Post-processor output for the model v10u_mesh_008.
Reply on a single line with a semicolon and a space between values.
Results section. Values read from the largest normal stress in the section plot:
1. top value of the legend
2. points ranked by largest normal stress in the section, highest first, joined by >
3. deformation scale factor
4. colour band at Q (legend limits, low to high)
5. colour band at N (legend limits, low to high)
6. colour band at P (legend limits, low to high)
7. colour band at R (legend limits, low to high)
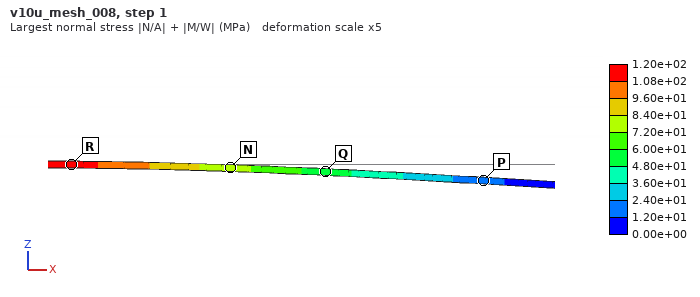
1.20e+02 MPa; R > N > Q > P; 5; 4.80e+01 to 6.00e+01 MPa; 7.20e+01 to 8.40e+01 MPa; 1.20e+01 to 2.40e+01 MPa; 1.08e+02 to 1.20e+02 MPa
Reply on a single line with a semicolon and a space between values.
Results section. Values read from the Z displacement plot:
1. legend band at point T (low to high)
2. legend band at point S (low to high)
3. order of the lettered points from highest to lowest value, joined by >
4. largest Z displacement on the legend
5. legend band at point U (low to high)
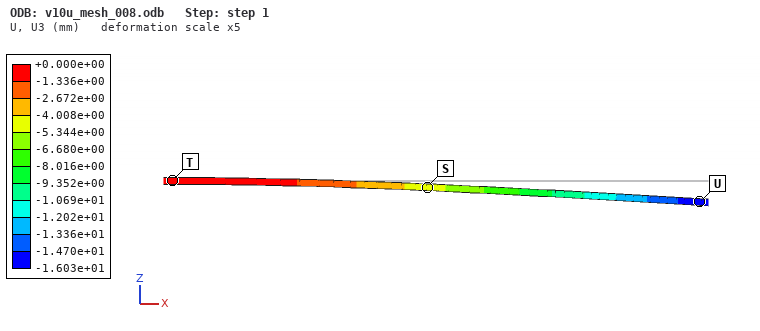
-1.336e+00 to +0.000e+00 mm; -5.344e+00 to -4.008e+00 mm; T > S > U; +0.000e+00 mm; -1.603e+01 to -1.470e+01 mm
